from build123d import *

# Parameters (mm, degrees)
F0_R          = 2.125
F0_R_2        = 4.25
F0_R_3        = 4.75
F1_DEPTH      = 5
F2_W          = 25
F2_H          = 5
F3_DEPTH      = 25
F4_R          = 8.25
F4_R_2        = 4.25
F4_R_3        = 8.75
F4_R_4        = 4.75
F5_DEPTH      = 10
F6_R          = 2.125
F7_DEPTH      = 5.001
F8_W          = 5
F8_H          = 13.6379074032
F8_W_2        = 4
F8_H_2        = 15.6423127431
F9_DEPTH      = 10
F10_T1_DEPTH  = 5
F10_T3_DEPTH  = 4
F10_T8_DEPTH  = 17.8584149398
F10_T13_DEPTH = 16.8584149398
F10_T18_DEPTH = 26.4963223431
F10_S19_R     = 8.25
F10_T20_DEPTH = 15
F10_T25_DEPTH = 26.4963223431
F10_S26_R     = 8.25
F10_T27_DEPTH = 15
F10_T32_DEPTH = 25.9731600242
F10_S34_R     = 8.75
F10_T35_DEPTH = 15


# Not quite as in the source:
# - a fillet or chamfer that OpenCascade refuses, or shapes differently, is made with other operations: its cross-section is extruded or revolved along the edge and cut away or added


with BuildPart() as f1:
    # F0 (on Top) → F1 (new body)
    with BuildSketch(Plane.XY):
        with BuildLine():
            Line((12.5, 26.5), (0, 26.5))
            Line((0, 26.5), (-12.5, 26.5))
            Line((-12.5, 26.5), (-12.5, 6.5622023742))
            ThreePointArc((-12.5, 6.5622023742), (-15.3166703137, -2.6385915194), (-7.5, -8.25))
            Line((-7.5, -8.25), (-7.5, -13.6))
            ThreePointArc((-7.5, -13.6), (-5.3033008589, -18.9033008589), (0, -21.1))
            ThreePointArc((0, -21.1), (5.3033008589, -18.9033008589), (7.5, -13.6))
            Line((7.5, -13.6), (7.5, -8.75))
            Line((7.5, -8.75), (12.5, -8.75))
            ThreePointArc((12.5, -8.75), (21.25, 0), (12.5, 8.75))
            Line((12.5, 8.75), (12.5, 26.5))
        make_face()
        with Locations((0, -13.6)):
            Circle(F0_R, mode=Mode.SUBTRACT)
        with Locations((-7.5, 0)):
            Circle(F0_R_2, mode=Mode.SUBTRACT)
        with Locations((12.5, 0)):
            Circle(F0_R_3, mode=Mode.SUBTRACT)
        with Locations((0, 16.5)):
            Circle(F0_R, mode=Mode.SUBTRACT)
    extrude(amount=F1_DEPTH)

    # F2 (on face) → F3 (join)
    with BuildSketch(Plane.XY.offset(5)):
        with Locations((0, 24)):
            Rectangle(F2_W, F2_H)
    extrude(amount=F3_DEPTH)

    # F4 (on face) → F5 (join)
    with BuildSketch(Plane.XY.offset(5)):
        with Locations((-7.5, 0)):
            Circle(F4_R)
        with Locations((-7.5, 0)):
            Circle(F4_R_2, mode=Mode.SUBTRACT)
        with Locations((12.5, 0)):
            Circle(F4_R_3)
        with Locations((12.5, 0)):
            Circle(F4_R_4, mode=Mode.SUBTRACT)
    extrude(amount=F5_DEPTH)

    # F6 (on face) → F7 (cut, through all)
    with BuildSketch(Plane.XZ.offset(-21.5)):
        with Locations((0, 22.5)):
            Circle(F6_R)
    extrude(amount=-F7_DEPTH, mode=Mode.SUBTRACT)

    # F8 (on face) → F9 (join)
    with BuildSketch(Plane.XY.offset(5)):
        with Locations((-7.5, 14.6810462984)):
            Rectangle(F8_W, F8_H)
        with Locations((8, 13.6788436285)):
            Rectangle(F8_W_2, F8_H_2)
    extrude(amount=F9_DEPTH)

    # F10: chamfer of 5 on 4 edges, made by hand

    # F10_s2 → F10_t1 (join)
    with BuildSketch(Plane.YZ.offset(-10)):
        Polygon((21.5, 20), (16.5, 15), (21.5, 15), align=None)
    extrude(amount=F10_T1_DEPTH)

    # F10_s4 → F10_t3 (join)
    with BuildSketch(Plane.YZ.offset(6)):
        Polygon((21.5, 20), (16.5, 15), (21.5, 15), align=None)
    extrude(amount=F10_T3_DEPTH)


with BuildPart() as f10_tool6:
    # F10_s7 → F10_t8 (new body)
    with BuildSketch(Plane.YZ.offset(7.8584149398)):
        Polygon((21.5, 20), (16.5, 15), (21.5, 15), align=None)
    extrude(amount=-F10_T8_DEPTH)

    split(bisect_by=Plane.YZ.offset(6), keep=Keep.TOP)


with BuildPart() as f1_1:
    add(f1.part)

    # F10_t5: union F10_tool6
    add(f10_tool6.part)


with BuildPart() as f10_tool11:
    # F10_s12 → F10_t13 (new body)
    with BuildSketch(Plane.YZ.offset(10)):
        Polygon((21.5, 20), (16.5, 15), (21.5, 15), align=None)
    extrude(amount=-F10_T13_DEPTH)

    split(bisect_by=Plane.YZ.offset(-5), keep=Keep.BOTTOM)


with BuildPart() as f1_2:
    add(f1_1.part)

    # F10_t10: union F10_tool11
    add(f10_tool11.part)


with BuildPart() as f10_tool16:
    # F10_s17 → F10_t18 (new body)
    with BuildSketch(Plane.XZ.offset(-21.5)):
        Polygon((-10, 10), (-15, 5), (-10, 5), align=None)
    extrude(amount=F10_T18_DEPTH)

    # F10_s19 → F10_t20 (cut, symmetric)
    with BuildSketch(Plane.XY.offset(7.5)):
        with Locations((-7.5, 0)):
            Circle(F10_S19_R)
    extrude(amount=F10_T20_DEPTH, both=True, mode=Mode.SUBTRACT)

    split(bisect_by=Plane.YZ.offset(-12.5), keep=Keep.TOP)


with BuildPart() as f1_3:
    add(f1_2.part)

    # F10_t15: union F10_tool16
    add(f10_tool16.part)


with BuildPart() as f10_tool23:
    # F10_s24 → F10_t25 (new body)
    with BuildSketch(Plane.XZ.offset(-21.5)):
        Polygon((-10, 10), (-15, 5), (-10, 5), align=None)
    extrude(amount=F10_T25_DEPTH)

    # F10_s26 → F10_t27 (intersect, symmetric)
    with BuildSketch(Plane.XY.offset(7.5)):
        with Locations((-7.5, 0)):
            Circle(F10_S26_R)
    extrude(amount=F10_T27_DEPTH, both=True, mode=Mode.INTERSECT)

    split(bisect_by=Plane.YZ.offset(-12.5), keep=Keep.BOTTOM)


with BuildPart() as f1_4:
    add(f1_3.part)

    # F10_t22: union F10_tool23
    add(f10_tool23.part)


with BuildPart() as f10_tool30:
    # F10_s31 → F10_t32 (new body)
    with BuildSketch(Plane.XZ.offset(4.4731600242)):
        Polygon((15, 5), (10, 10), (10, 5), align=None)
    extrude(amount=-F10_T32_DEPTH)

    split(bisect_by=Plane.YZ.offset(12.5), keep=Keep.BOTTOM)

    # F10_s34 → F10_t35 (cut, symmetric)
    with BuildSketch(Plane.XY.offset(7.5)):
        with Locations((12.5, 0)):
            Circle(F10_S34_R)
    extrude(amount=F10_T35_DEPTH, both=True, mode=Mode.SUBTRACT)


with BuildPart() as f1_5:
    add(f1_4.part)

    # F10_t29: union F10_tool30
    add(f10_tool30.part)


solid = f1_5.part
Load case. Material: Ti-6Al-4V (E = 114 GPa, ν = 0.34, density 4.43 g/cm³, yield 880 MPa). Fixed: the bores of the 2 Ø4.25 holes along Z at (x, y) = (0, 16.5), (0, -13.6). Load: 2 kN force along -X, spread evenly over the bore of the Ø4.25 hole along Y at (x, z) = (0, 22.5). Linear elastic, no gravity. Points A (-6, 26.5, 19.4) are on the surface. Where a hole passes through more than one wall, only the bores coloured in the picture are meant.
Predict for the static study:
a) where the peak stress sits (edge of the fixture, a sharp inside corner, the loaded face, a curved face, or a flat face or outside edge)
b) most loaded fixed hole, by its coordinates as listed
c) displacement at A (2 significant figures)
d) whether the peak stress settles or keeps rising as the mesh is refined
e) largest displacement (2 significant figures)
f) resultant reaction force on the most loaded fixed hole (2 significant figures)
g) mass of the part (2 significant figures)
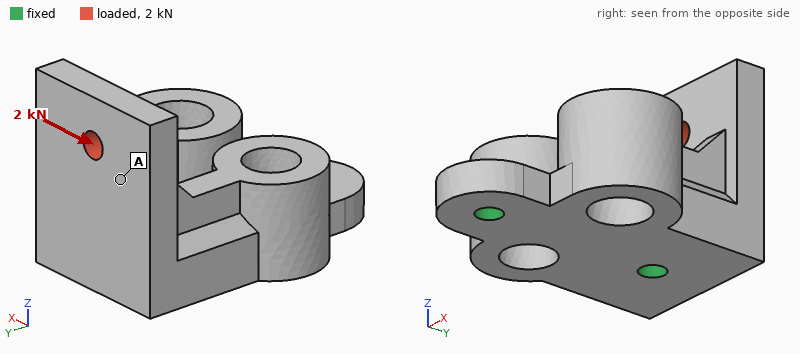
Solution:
edge of the fixture
(0, 16.5)
0.076 mm
keeps rising
0.13 mm
2.3 kN
58 g
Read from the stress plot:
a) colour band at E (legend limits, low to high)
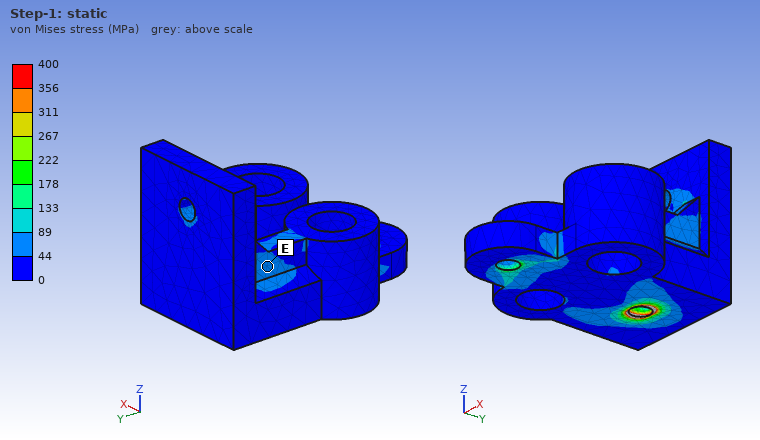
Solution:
44 to 89 MPa
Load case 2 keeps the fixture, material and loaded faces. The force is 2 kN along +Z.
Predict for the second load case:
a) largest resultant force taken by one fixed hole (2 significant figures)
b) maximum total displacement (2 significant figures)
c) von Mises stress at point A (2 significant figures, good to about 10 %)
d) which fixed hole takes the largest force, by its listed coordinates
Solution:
2.4 kN
21 µm
18 MPa
(0, 16.5)
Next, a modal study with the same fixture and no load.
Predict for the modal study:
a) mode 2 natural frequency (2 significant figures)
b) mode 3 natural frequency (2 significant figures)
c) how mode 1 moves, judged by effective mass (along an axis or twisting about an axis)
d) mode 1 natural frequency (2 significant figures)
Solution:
9200 Hz
11 kHz
along X
5600 Hz
